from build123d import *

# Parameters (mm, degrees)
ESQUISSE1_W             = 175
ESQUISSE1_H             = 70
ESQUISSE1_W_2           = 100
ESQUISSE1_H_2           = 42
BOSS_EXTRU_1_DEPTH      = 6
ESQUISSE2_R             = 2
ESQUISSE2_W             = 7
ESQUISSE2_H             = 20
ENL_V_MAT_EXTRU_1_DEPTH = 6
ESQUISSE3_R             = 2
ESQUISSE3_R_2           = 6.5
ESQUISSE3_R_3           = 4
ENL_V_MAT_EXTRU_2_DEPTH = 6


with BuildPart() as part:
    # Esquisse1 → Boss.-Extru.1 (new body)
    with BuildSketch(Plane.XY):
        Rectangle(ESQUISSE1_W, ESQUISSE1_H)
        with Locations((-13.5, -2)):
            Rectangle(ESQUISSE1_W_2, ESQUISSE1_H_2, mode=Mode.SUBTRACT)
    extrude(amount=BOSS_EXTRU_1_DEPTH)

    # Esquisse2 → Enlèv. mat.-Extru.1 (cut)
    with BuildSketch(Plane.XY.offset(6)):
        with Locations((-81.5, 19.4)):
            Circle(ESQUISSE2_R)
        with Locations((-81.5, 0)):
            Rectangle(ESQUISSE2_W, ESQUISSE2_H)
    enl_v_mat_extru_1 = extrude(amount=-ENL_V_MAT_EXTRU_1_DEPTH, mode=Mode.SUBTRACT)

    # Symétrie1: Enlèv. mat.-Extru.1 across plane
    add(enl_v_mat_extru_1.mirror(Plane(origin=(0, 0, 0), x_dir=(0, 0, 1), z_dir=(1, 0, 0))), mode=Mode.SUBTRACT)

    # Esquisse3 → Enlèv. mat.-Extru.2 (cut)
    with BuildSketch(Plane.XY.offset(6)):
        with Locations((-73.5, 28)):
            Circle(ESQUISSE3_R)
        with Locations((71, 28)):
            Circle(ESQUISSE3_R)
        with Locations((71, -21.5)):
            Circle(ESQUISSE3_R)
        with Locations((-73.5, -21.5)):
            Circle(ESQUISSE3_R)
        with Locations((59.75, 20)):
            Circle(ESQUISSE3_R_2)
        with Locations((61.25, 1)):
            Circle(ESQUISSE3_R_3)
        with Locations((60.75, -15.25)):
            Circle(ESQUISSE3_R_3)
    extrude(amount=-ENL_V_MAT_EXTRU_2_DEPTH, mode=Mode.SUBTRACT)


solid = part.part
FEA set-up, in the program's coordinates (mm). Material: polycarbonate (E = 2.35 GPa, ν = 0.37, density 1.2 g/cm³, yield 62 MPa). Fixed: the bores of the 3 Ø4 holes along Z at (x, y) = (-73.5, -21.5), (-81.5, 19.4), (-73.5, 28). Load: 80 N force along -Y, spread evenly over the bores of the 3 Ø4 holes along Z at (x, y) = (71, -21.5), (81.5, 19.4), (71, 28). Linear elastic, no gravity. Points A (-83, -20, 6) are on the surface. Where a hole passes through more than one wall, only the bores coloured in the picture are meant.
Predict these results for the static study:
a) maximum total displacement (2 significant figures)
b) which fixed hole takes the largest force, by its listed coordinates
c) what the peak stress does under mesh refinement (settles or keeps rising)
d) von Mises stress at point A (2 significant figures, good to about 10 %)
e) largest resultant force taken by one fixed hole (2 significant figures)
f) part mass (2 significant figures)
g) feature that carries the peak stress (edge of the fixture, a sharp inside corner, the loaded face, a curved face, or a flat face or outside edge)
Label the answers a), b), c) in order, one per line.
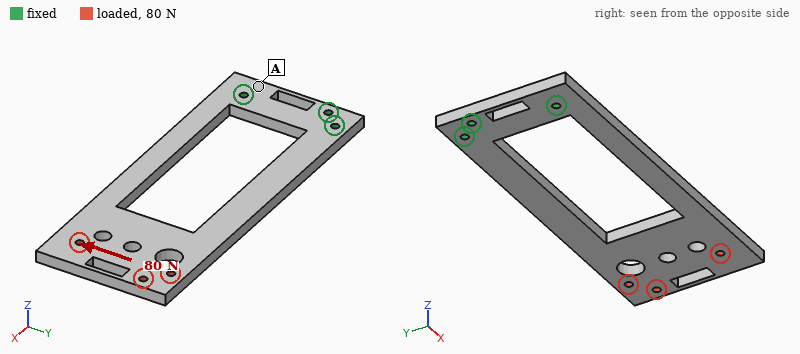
a) 2.0 mm
b) (-73.5, 28)
c) keeps rising
d) 1.7 MPa
e) 300 N
f) 54 g
g) edge of the fixture
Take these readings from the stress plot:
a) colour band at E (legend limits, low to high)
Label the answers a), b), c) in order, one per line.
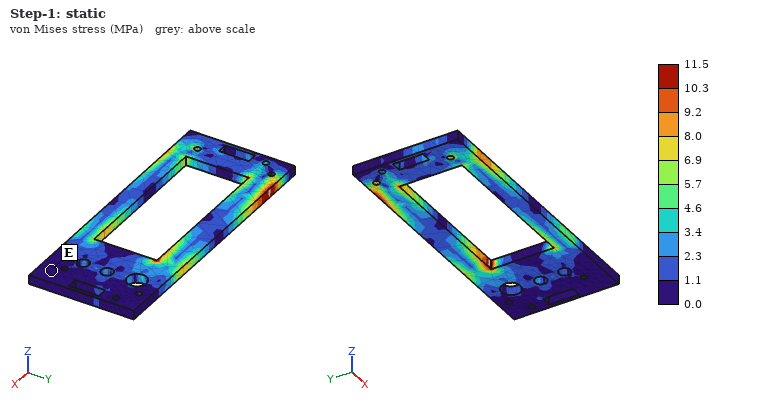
a) 0.0 to 1.1 MPa
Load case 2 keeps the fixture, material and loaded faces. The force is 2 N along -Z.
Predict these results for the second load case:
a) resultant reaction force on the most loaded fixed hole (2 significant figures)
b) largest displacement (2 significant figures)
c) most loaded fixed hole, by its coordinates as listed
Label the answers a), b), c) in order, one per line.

a) 5.4 N
b) 2.0 mm
c) (-73.5, 28)
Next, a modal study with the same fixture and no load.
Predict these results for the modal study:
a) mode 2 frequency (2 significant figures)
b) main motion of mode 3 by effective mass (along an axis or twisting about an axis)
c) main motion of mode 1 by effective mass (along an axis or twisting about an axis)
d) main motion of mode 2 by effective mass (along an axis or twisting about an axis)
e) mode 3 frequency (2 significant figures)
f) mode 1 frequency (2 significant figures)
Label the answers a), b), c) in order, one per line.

a) 160 Hz
b) along Y
c) along Z
d) twisting about X
e) 190 Hz
f) 38 Hz
